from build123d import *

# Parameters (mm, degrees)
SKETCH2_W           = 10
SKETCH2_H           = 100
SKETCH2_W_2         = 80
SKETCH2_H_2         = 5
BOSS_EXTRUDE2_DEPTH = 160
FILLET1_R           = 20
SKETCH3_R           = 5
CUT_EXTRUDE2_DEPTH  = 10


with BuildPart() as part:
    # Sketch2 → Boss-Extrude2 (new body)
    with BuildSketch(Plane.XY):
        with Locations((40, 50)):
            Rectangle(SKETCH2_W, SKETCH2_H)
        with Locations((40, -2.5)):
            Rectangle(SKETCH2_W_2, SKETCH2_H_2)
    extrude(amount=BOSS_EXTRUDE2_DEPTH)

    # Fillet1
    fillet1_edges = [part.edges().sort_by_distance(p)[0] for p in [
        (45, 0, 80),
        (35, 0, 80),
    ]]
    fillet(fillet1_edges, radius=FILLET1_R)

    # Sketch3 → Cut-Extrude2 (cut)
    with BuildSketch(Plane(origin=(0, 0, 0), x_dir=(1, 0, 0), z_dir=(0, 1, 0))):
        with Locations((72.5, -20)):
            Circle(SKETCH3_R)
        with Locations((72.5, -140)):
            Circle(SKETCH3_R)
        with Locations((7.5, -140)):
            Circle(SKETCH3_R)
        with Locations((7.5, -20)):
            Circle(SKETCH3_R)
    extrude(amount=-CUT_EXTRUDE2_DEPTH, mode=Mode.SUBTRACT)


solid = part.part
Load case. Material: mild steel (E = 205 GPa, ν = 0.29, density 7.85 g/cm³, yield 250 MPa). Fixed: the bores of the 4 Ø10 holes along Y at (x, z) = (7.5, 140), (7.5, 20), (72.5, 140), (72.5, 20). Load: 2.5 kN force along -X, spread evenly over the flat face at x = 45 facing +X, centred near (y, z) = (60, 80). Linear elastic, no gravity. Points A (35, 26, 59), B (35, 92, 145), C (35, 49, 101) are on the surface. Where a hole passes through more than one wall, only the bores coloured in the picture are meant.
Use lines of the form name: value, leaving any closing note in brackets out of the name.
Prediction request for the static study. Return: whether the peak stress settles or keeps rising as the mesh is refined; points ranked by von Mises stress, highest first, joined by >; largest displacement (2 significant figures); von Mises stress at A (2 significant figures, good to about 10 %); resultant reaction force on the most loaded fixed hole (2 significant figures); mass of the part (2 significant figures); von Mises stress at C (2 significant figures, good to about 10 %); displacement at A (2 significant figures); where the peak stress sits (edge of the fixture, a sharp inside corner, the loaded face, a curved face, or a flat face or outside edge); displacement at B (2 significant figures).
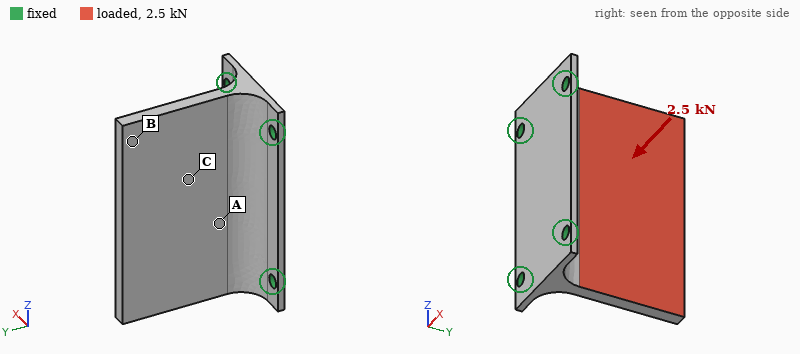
whether the peak stress settles or keeps rising as the mesh is refined: keeps rising
points ranked by von Mises stress, highest first, joined by >: A > C > B
largest displacement: 0.14 mm
von Mises stress at A: 26 MPa
resultant reaction force on the most loaded fixed hole: 1.7 kN
mass of the part: 2.0 kg
von Mises stress at C: 14 MPa
displacement at A: 0.022 mm
where the peak stress sits: edge of the fixture
displacement at B: 0.12 mm
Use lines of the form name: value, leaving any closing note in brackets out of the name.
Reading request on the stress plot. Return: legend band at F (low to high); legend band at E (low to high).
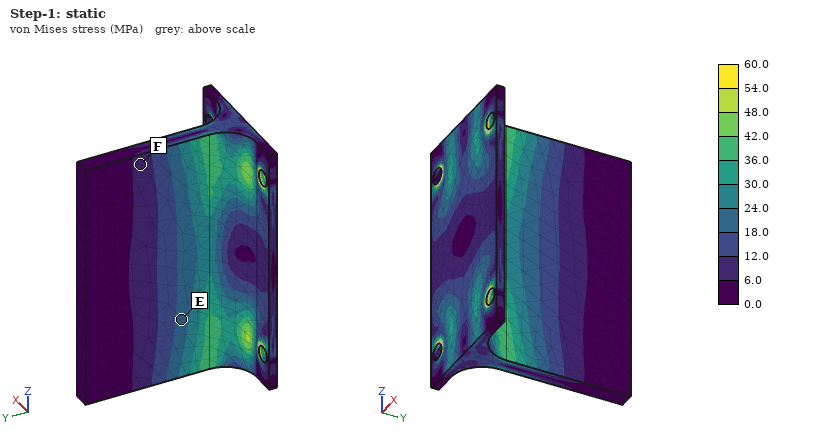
legend band at F: 6.0 to 12.0 MPa
legend band at E: 18.0 to 24.0 MPa
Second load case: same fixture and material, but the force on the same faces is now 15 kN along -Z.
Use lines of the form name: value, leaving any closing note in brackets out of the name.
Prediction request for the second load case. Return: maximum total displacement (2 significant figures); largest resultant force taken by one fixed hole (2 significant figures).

maximum total displacement: 80 µm
largest resultant force taken by one fixed hole: 6.8 kN
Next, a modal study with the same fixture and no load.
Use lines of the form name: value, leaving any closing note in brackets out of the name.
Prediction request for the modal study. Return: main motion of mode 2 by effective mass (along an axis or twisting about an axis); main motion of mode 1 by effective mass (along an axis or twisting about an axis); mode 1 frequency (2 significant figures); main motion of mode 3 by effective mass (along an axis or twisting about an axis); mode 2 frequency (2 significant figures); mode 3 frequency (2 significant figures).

main motion of mode 2 by effective mass: twisting about Y
main motion of mode 1 by effective mass: along X
mode 1 frequency: 830 Hz
main motion of mode 3 by effective mass: along Z
mode 2 frequency: 1600 Hz
mode 3 frequency: 2500 Hz
